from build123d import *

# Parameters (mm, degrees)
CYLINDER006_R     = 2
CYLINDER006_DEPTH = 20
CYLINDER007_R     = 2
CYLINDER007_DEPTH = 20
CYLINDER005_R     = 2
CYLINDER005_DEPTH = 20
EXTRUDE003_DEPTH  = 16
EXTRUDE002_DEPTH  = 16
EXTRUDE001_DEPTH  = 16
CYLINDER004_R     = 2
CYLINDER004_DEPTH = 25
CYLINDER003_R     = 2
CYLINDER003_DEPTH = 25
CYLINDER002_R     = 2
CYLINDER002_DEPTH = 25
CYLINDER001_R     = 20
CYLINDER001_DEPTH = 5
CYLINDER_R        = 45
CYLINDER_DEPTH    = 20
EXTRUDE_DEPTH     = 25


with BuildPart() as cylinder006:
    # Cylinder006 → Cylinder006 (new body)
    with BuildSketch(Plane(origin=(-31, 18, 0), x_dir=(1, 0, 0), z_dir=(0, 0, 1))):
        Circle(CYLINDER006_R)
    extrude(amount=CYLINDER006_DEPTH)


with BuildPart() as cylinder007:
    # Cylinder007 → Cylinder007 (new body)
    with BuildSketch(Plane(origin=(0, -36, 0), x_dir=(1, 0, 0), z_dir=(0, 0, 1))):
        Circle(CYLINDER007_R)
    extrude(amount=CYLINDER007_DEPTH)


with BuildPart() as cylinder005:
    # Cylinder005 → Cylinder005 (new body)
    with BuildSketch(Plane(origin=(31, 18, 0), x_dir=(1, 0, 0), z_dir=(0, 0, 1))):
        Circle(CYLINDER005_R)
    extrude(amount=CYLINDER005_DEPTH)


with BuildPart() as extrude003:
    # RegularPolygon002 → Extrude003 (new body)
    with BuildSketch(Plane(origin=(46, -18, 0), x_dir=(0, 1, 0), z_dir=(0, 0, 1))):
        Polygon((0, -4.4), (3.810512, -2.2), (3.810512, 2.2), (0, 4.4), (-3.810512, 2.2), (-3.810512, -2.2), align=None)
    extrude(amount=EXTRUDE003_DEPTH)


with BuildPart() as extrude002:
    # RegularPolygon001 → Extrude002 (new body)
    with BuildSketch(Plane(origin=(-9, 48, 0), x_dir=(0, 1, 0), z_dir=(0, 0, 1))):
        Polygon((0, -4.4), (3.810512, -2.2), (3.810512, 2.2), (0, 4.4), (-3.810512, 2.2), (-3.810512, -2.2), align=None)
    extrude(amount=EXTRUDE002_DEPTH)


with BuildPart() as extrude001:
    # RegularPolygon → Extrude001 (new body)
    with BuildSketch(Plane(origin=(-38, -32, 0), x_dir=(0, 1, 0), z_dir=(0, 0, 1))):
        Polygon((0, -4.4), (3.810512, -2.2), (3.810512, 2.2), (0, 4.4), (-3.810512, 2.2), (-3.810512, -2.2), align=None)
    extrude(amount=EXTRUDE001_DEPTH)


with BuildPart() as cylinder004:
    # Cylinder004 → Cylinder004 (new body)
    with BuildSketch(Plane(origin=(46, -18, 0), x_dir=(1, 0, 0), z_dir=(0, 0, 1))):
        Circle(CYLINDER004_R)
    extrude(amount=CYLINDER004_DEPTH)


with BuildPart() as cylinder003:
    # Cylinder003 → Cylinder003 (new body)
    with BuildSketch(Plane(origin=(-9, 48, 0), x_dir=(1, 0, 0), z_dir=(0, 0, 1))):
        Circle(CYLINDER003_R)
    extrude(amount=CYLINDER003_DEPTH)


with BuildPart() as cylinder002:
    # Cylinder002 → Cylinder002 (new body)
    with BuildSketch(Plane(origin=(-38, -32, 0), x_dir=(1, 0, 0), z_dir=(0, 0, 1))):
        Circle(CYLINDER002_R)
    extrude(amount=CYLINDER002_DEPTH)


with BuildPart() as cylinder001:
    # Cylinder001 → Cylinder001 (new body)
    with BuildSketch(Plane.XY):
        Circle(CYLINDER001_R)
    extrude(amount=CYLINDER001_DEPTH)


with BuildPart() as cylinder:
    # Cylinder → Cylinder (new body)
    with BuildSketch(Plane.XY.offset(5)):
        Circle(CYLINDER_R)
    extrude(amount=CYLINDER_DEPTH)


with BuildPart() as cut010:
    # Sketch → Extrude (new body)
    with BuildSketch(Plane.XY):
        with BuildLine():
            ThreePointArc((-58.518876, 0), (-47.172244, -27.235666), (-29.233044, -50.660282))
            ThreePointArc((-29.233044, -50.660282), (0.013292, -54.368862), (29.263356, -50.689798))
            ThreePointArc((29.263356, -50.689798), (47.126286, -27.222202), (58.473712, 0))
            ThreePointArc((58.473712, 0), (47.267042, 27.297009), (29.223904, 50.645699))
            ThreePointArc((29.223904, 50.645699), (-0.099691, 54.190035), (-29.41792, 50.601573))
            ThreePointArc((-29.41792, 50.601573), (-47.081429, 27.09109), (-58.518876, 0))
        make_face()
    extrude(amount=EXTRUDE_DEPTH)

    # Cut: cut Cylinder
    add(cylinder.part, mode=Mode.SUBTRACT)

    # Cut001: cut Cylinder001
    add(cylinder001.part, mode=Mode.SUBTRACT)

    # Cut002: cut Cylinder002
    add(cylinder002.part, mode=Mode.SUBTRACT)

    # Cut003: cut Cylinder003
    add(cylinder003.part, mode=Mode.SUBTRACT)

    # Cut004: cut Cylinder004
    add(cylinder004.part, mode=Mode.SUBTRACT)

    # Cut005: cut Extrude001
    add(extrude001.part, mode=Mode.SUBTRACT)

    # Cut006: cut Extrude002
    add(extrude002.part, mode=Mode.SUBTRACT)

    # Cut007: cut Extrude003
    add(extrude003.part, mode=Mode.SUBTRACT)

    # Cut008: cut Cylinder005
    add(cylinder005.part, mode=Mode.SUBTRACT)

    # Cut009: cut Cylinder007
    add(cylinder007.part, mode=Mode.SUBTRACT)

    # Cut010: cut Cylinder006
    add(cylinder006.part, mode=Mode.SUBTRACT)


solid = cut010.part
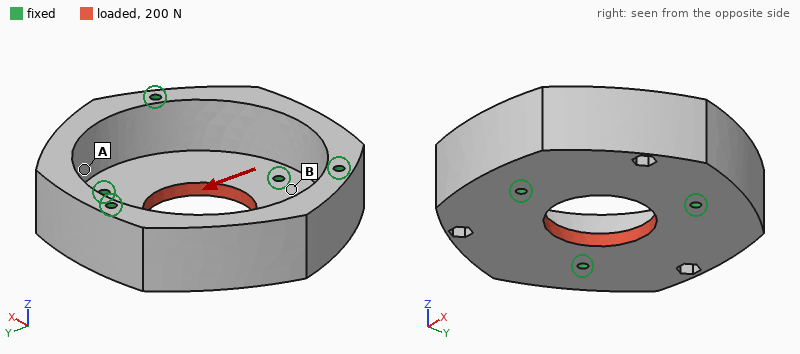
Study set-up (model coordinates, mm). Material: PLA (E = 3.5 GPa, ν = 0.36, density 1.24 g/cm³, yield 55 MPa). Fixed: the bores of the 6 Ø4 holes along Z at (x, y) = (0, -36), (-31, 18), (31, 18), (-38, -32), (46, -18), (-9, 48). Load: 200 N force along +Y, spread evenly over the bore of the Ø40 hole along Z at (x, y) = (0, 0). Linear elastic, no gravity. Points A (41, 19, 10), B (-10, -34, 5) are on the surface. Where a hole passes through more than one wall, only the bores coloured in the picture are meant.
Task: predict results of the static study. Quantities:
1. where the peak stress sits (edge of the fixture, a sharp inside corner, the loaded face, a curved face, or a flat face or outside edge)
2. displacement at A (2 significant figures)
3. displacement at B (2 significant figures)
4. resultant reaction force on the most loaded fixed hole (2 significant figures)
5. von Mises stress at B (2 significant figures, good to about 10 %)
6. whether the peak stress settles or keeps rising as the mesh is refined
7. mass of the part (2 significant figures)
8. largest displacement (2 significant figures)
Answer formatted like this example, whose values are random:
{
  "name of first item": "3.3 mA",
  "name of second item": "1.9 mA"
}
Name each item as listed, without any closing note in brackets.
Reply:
{
  "where the peak stress sits": "edge of the fixture",
  "displacement at A": "0.93 µm",
  "displacement at B": "1.6 µm",
  "resultant reaction force on the most loaded fixed hole": "60 N",
  "von Mises stress at B": "0.23 MPa",
  "whether the peak stress settles or keeps rising as the mesh is refined": "keeps rising",
  "mass of the part": "130 g",
  "largest displacement": "6.1 µm"
}
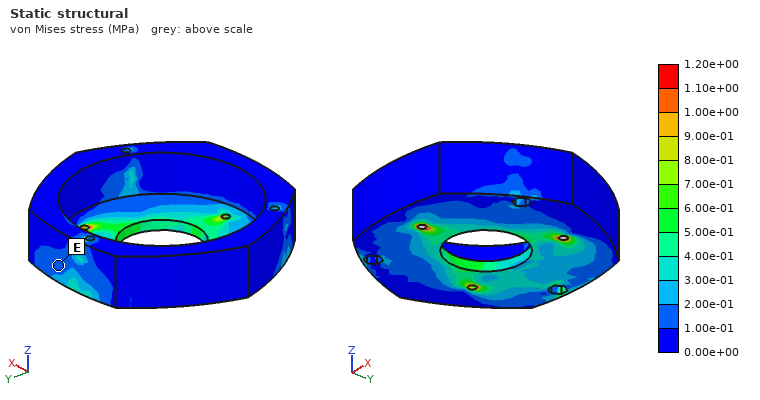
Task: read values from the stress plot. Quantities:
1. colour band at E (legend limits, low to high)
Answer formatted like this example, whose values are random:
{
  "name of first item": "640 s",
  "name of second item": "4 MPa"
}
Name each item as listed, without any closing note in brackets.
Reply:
{
  "colour band at E": "1.00e-01 to 2.00e-01 MPa"
}
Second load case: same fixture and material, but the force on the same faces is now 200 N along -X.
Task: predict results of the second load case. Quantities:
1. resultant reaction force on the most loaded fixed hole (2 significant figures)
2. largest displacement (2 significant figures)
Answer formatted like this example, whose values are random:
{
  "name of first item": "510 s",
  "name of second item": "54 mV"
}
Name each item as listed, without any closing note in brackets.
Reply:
{
  "resultant reaction force on the most loaded fixed hole": "60 N",
  "largest displacement": "5.5 µm"
}
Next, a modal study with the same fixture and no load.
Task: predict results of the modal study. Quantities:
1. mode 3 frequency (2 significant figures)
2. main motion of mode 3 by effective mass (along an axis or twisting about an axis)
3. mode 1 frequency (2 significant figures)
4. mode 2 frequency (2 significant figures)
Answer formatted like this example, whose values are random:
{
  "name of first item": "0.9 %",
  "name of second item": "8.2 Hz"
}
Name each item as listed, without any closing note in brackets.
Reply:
{
  "mode 3 frequency": "3000 Hz",
  "main motion of mode 3 by effective mass": "along Z",
  "mode 1 frequency": "2700 Hz",
  "mode 2 frequency": "2800 Hz"
}
